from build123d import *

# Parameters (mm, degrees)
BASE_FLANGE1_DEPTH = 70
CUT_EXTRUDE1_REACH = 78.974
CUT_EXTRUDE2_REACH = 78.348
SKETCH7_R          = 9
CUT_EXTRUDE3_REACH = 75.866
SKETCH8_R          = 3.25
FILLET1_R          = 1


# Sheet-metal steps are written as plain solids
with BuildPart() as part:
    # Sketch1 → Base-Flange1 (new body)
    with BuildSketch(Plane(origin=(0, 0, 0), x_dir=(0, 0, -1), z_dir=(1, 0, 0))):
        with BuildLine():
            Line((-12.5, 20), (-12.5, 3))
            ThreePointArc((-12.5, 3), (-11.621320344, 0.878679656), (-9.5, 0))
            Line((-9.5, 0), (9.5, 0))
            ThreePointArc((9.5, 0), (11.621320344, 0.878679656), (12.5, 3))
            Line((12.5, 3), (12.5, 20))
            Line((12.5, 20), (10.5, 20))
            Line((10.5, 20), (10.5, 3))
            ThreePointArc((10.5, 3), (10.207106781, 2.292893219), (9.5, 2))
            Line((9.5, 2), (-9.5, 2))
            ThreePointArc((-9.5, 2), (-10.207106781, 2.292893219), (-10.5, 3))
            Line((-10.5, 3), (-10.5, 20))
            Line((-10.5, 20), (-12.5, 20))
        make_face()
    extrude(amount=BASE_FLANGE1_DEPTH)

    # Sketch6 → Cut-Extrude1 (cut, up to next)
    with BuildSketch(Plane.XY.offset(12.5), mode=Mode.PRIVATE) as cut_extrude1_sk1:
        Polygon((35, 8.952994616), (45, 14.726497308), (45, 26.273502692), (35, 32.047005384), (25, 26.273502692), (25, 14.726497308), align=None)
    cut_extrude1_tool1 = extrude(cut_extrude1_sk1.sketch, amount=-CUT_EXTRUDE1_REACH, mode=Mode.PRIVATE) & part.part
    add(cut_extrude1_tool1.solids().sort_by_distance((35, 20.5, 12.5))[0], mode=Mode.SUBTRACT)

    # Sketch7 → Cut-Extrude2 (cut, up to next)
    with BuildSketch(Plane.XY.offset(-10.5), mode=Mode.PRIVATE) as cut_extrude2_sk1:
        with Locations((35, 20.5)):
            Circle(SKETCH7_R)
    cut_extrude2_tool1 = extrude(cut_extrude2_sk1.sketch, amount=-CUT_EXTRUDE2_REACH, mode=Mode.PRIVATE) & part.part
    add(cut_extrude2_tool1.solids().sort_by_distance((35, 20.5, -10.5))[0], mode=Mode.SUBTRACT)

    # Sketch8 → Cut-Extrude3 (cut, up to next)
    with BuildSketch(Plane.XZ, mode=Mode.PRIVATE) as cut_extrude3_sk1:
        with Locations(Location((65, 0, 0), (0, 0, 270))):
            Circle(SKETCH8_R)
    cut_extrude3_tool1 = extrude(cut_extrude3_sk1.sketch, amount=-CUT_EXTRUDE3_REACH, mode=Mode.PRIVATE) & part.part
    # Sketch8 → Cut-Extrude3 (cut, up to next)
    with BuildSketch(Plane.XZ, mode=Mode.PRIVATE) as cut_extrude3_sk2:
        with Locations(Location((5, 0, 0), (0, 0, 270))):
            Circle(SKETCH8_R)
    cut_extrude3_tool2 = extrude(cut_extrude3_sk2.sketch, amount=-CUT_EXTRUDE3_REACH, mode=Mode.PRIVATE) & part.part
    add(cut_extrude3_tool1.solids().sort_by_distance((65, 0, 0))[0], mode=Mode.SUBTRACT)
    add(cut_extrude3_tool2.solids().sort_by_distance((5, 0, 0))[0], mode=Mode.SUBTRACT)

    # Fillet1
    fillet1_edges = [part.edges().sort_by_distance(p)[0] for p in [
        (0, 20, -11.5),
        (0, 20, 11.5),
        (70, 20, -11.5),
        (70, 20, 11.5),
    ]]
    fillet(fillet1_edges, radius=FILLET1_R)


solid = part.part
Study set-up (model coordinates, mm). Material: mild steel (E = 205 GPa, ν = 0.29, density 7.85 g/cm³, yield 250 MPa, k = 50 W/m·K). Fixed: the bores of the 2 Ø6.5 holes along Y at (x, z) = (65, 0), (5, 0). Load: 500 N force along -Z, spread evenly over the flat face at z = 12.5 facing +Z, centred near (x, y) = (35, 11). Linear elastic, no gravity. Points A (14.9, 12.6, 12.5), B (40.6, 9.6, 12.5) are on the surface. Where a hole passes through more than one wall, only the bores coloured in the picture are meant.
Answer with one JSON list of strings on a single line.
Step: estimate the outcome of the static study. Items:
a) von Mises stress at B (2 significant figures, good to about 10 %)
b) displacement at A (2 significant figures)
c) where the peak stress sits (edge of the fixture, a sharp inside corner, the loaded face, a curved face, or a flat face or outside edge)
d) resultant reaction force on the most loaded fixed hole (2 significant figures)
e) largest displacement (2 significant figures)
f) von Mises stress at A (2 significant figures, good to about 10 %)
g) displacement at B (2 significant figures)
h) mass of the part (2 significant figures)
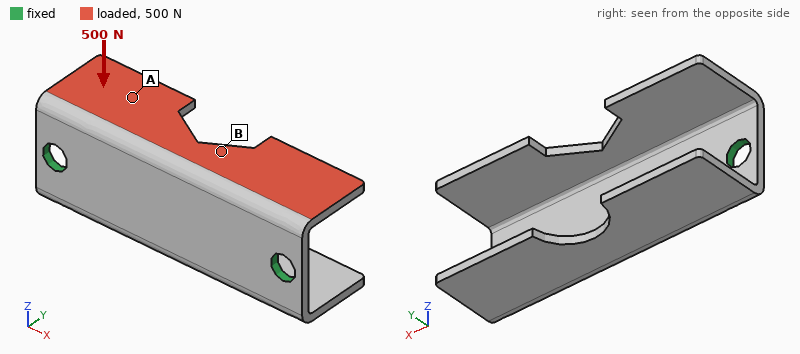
["40 MPa", "0.095 mm", "a flat face or outside edge", "250 N", "0.16 mm", "17 MPa", "0.070 mm", "60 g"]
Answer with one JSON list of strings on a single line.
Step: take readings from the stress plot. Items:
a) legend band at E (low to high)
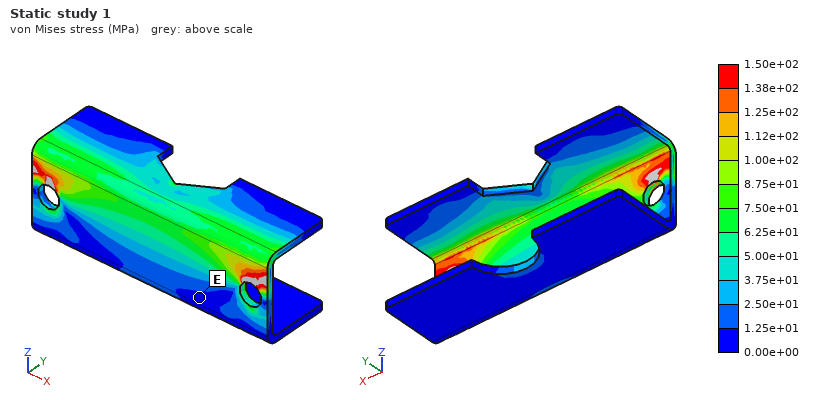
["0.00e+00 to 1.25e+01 MPa"]
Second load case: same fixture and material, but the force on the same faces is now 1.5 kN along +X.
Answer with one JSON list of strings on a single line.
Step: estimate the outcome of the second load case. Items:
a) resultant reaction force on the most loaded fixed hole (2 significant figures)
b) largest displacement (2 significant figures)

["840 N", "46 µm"]
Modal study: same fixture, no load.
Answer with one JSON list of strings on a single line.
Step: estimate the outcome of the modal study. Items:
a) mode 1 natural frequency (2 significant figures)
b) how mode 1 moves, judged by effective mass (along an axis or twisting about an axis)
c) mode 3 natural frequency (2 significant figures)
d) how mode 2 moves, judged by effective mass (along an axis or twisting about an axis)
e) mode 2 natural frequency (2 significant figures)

["2400 Hz", "along Z", "3300 Hz", "along Y", "2800 Hz"]
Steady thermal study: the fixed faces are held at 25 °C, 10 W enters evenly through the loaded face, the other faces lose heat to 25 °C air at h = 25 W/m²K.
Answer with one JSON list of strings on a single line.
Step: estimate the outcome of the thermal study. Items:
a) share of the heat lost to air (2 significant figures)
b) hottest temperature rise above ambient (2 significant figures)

["23 %", "34 K"]
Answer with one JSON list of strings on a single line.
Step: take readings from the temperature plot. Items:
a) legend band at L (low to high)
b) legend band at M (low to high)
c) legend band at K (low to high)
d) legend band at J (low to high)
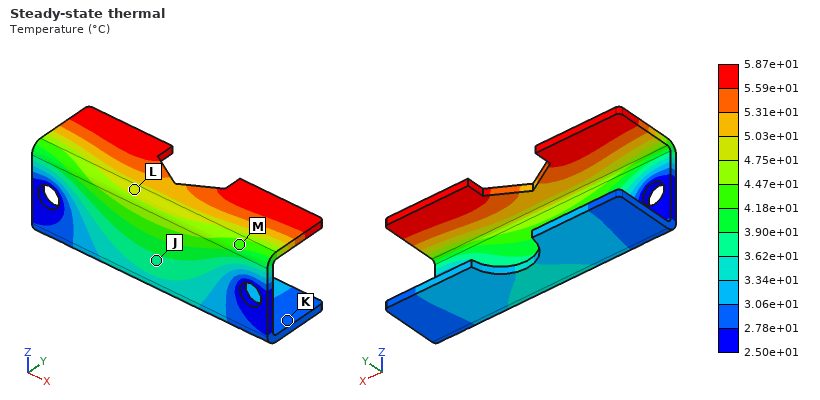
["4.75e+01 to 5.03e+01 °C", "4.18e+01 to 4.47e+01 °C", "2.78e+01 to 3.06e+01 °C", "3.62e+01 to 3.90e+01 °C"]
